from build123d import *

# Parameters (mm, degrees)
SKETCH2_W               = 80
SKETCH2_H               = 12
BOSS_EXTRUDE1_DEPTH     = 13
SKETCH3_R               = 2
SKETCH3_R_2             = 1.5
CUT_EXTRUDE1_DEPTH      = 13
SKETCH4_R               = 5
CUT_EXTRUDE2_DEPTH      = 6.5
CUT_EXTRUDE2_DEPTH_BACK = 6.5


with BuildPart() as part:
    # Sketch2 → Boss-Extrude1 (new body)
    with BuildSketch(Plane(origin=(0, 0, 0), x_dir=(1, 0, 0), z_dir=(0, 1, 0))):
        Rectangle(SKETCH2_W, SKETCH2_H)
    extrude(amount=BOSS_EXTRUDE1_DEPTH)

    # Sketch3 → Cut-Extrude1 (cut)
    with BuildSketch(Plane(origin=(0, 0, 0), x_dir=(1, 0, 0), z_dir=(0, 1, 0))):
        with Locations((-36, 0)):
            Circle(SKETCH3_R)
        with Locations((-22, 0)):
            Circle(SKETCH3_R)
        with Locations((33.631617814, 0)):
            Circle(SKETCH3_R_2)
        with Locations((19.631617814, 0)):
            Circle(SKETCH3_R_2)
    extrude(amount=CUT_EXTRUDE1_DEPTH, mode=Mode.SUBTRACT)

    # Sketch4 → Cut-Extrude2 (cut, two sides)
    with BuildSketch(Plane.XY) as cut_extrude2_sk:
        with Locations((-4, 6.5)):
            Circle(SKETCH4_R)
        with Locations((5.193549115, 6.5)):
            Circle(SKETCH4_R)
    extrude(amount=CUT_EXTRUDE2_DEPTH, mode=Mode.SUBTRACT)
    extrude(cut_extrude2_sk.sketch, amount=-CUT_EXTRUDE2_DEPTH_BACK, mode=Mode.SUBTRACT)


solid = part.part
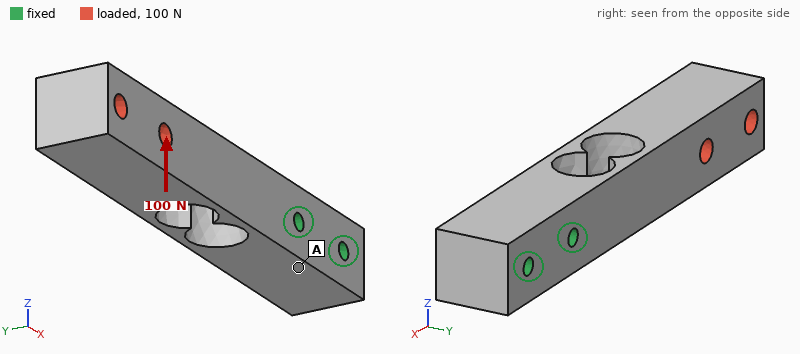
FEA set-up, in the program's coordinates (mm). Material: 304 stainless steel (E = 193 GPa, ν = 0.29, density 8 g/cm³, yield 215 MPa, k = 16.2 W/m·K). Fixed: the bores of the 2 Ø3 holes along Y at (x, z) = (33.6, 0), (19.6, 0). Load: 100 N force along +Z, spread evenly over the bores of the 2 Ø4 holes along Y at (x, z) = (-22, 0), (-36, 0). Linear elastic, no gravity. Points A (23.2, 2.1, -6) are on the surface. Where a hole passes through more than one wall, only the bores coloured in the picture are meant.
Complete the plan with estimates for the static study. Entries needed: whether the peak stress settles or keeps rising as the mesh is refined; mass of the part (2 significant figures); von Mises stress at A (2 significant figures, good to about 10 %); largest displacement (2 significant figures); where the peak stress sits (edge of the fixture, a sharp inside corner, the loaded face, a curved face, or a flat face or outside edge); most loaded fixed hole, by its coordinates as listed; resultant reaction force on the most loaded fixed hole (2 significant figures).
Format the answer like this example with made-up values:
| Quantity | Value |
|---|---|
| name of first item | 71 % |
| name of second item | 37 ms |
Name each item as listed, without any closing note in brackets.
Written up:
| Quantity | Value |
|---|---|
| whether the peak stress settles or keeps rising as the mesh is refined | keeps rising |
| mass of the part | 81 g |
| von Mises stress at A | 8.0 MPa |
| largest displacement | 39 µm |
| where the peak stress sits | a sharp inside corner |
| most loaded fixed hole, by its coordinates as listed | (19.6, 0) |
| resultant reaction force on the most loaded fixed hole | 320 N |
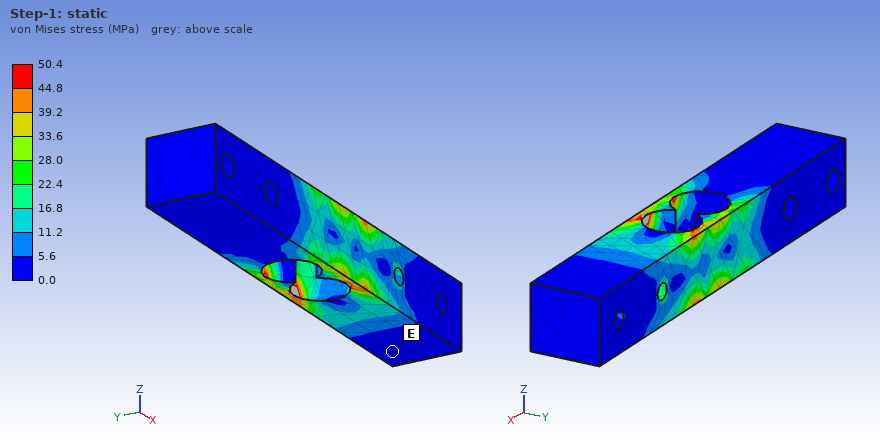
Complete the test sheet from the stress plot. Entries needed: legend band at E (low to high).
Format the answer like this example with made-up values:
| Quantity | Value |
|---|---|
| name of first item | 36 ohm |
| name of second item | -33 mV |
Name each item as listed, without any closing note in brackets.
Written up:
| Quantity | Value |
|---|---|
| legend band at E | 0.0 to 5.6 MPa |
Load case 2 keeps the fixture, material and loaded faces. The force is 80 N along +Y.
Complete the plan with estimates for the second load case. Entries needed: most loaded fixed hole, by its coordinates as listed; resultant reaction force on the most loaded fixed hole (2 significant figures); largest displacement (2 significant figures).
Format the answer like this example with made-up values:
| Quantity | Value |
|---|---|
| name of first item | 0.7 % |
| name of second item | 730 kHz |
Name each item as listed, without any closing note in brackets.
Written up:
| Quantity | Value |
|---|---|
| most loaded fixed hole, by its coordinates as listed | (19.6, 0) |
| resultant reaction force on the most loaded fixed hole | 120 N |
| largest displacement | 28 µm |
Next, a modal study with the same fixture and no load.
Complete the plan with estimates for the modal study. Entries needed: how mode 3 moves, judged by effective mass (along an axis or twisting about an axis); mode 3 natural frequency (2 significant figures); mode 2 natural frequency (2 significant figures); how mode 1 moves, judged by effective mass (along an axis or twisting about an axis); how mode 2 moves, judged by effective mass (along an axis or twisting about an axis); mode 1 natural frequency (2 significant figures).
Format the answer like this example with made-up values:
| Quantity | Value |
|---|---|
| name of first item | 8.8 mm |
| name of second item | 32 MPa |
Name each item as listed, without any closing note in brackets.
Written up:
| Quantity | Value |
|---|---|
| how mode 3 moves, judged by effective mass | twisting about X |
| mode 3 natural frequency | 6500 Hz |
| mode 2 natural frequency | 1700 Hz |
| how mode 1 moves, judged by effective mass | along Y |
| how mode 2 moves, judged by effective mass | along Z |
| mode 1 natural frequency | 1500 Hz |
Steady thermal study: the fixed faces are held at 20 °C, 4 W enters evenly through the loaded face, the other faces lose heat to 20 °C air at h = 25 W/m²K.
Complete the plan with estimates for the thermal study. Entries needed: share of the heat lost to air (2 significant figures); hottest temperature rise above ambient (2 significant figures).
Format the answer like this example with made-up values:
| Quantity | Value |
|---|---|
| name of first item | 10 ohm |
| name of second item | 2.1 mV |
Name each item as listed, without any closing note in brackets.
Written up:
| Quantity | Value |
|---|---|
| share of the heat lost to air | 71 % |
| hottest temperature rise above ambient | 60 K |
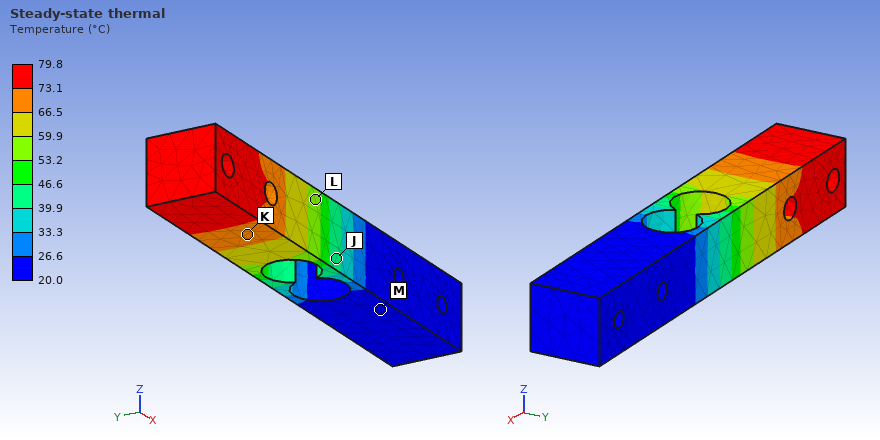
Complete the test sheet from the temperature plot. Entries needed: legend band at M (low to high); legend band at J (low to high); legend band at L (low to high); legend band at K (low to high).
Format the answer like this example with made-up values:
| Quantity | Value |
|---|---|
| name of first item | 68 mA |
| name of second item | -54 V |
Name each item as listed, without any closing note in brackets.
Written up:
| Quantity | Value |
|---|---|
| legend band at M | 20.0 to 26.6 °C |
| legend band at J | 39.9 to 46.6 °C |
| legend band at L | 53.2 to 59.9 °C |
| legend band at K | 66.5 to 73.1 °C |
